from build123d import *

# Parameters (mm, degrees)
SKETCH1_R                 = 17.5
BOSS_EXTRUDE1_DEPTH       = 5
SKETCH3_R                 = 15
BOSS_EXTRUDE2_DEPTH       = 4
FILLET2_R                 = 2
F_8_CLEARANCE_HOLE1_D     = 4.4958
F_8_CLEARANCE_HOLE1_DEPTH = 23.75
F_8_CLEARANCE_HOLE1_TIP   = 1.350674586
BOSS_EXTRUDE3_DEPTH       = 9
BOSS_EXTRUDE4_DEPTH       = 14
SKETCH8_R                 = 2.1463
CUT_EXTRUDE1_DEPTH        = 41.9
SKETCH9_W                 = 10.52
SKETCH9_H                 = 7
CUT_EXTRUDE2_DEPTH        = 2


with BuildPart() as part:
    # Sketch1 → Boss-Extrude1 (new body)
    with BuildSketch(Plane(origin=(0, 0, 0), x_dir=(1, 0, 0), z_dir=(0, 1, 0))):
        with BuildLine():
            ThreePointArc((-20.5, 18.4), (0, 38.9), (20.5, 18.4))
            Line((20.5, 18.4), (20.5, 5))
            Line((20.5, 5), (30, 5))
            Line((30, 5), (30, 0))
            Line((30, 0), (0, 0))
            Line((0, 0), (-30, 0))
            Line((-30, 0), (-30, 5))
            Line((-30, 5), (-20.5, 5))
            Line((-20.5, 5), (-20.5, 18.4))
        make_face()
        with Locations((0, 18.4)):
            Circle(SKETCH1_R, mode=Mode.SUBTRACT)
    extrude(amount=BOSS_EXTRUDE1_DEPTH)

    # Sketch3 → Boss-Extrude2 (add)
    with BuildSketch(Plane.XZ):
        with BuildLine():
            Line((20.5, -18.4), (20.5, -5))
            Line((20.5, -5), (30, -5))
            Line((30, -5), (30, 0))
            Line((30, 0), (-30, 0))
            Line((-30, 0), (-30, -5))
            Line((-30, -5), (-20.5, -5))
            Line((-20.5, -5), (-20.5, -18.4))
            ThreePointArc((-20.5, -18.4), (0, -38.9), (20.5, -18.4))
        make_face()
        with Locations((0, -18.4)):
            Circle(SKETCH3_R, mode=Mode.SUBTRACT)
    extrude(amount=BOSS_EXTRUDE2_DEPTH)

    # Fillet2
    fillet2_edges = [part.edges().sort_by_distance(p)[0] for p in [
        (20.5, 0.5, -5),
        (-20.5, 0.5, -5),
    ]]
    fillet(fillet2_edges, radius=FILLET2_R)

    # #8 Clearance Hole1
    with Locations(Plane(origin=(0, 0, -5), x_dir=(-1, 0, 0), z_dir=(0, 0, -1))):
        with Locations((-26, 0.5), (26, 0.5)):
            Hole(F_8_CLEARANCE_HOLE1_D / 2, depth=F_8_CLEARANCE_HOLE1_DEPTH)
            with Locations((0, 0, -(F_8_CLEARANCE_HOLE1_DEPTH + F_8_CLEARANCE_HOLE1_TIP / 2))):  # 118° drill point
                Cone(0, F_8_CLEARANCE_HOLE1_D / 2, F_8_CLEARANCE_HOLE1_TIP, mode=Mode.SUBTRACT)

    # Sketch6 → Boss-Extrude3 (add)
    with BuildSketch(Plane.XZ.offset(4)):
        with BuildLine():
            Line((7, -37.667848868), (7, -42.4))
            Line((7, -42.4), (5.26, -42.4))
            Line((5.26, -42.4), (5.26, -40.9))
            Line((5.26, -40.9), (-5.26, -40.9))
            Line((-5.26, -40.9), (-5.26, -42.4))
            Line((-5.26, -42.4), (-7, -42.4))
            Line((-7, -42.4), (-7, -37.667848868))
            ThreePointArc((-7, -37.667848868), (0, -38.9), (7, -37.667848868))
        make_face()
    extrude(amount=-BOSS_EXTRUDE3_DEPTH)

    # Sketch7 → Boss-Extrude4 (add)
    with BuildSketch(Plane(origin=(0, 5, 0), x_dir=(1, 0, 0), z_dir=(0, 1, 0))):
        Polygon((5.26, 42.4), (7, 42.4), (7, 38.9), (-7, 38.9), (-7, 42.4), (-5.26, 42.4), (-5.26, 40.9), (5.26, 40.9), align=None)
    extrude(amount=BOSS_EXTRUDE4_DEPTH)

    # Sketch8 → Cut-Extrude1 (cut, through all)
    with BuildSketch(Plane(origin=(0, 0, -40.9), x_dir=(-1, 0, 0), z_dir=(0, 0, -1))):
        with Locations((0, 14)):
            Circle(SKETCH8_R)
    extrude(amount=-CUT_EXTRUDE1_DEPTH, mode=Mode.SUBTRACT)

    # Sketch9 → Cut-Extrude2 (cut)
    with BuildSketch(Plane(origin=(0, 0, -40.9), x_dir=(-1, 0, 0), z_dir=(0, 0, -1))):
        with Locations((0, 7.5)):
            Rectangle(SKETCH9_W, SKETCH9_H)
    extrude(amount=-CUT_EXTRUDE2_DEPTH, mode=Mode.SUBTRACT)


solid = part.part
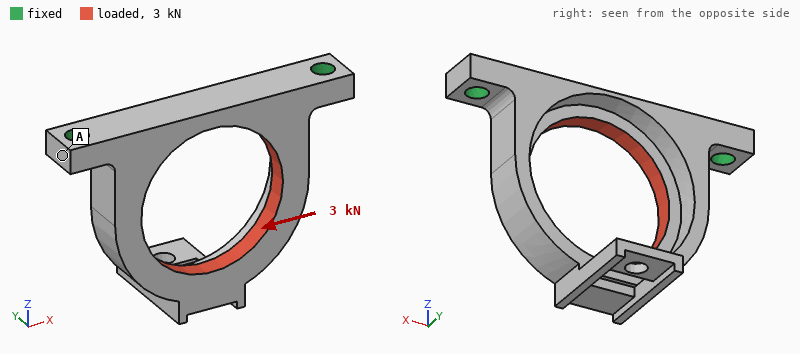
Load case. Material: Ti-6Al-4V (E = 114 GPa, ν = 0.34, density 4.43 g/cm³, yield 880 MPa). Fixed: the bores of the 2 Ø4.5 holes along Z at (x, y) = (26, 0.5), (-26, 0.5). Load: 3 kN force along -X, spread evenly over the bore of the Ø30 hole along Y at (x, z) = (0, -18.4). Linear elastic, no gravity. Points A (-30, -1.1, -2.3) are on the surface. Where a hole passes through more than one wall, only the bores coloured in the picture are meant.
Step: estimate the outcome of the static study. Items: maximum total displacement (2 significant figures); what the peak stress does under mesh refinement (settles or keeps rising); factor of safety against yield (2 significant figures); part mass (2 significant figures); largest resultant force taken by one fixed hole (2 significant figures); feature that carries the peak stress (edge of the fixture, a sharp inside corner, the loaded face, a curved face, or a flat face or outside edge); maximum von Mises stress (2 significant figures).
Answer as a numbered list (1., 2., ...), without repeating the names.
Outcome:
1. 0.15 mm
2. settles
3. 3.5
4. 29 g
5. 1.8 kN
6. a curved face
7. 250 MPa
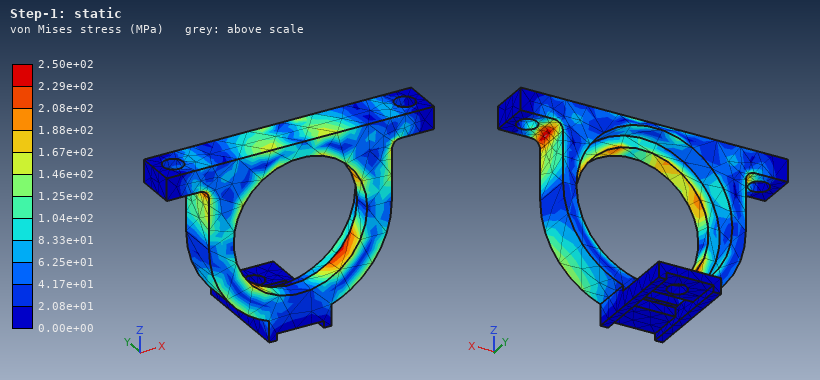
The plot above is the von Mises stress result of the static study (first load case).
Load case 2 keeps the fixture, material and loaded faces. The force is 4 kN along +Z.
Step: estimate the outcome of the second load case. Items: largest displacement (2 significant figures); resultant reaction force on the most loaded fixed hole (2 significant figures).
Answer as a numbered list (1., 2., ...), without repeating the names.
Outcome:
1. 0.17 mm
2. 2.0 kN
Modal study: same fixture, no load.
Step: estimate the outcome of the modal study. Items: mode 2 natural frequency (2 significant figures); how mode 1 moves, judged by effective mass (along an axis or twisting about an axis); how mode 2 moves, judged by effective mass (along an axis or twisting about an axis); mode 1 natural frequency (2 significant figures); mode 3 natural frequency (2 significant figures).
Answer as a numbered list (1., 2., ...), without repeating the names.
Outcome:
1. 4500 Hz
2. along Y
3. along X
4. 2300 Hz
5. 6100 Hz
